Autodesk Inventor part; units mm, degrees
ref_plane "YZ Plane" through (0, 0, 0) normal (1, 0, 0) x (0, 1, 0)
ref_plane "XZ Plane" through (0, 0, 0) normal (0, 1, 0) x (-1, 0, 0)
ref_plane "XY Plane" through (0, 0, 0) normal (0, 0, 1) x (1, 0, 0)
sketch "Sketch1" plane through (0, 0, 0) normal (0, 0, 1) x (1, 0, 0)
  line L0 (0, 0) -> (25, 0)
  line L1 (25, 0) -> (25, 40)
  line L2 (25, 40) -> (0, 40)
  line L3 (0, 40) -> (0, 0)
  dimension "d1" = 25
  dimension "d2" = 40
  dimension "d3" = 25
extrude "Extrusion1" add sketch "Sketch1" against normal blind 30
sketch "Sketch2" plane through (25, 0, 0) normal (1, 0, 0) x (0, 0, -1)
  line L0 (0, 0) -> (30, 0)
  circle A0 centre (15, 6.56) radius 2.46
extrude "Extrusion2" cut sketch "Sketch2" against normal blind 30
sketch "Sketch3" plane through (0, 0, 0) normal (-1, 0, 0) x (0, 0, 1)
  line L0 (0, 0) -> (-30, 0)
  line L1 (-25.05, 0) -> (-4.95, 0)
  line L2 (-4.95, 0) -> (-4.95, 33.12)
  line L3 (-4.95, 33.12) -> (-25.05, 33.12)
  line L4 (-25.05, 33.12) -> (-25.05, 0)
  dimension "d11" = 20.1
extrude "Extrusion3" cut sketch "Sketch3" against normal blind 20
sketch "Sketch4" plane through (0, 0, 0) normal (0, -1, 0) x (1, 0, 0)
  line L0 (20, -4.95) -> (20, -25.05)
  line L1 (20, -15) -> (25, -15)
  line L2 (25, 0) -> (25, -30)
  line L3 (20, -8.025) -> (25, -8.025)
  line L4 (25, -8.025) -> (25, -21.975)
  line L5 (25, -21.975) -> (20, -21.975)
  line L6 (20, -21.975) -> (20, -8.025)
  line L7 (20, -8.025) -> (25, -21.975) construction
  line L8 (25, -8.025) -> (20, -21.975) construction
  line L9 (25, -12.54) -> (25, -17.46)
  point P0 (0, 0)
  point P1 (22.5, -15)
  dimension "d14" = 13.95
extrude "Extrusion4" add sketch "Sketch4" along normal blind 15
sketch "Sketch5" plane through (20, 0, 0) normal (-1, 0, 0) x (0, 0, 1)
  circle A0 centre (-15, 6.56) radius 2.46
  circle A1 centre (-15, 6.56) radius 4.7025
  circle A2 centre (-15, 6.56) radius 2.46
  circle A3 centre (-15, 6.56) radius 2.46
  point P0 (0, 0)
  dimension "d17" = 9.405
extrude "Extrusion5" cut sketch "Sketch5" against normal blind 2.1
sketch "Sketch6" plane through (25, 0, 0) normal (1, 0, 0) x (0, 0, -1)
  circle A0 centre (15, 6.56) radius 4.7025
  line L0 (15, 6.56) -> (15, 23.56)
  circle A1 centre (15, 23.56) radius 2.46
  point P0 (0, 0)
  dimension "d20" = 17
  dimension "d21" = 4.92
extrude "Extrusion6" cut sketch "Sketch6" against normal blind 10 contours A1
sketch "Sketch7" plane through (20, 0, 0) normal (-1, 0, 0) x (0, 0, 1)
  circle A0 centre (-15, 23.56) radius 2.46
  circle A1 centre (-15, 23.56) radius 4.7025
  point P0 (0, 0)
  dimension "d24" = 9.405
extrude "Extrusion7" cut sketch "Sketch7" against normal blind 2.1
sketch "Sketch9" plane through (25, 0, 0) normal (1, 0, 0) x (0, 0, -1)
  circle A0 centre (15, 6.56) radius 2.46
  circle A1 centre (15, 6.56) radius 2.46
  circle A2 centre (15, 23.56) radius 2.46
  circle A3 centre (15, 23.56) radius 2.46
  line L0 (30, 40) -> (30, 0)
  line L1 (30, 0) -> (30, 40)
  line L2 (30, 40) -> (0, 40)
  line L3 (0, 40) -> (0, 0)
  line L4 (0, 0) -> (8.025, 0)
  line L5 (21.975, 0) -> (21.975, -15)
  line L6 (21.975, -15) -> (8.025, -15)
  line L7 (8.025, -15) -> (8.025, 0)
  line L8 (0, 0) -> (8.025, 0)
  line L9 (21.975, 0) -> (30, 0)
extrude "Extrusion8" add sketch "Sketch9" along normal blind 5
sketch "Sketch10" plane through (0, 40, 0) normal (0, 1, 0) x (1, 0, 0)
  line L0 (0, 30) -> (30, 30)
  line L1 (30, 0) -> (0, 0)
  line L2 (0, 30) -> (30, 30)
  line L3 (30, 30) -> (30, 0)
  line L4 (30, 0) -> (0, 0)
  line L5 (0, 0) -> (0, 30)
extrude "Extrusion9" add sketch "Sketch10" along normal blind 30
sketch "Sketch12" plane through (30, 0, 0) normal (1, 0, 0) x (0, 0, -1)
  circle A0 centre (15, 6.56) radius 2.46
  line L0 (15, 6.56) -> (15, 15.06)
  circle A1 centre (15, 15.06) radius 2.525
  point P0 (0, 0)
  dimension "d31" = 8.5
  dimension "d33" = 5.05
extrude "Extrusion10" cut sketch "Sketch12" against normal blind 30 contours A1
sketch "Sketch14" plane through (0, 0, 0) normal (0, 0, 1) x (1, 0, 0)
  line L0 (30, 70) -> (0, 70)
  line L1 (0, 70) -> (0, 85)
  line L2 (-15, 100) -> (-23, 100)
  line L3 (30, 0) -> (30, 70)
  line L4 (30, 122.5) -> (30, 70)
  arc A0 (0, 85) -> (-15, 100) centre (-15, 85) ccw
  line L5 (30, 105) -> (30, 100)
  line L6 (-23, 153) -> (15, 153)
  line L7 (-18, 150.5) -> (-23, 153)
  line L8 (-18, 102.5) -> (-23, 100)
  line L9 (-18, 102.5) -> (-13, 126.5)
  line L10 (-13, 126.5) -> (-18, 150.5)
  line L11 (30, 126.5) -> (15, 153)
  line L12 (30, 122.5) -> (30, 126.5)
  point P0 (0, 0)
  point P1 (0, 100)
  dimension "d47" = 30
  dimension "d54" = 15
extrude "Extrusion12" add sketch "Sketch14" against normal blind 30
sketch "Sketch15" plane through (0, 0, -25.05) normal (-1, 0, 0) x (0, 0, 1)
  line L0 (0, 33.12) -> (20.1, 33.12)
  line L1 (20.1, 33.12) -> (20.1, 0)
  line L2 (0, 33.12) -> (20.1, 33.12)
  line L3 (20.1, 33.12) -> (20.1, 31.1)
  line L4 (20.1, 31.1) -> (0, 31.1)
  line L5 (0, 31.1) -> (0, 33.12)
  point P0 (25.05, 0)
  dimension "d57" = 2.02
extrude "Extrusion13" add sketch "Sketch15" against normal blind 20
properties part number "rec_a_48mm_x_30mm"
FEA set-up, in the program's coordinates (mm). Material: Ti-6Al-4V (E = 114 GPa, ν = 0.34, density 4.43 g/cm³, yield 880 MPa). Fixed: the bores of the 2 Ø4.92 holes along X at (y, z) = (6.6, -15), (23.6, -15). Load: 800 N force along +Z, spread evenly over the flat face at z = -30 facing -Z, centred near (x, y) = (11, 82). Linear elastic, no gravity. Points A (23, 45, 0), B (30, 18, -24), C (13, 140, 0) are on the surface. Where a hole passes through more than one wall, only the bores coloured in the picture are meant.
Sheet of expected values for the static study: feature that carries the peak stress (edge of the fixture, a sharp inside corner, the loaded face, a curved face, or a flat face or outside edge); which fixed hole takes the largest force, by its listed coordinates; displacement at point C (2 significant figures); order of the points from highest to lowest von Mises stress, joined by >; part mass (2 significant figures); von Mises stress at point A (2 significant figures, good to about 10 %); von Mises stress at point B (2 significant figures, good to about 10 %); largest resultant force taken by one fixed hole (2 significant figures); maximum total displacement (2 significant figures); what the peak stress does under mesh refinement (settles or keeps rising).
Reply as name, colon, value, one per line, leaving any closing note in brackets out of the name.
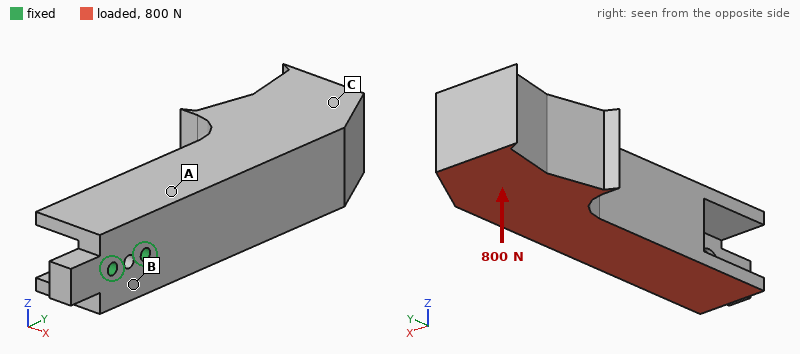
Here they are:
feature that carries the peak stress: edge of the fixture
which fixed hole takes the largest force, by its listed coordinates: (23.6, -15)
displacement at point C: 72 µm
order of the points from highest to lowest von Mises stress, joined by >: B > A > C
part mass: 650 g
von Mises stress at point A: 9.0 MPa
von Mises stress at point B: 17 MPa
largest resultant force taken by one fixed hole: 2.8 kN
maximum total displacement: 89 µm
what the peak stress does under mesh refinement: keeps rising
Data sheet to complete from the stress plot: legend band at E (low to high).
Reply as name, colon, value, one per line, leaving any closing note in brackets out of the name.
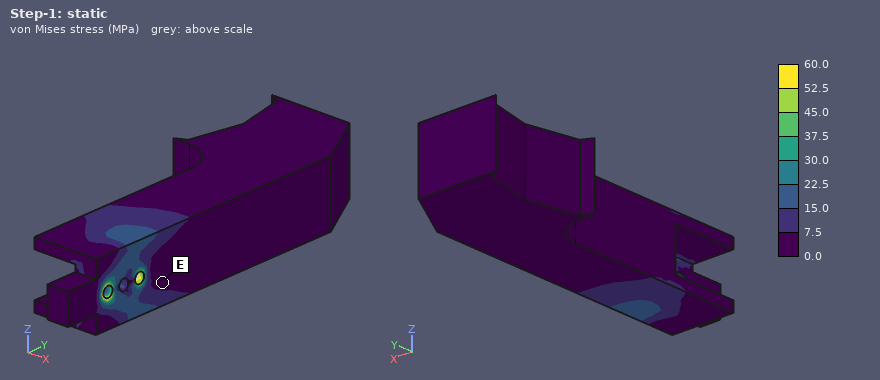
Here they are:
legend band at E: 0.0 to 7.5 MPa
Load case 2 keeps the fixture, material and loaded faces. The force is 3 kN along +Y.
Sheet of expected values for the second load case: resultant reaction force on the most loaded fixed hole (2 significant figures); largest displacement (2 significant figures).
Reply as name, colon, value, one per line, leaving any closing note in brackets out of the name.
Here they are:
resultant reaction force on the most loaded fixed hole: 3.1 kN
largest displacement: 0.12 mm
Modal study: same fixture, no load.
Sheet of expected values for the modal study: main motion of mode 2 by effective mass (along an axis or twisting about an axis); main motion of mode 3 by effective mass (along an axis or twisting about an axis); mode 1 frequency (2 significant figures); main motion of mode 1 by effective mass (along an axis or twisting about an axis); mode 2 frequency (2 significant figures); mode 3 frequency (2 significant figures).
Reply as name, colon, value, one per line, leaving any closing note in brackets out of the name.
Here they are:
main motion of mode 2 by effective mass: along Z
main motion of mode 3 by effective mass: twisting about Y
mode 1 frequency: 610 Hz
main motion of mode 1 by effective mass: along X
mode 2 frequency: 720 Hz
mode 3 frequency: 2300 Hz
